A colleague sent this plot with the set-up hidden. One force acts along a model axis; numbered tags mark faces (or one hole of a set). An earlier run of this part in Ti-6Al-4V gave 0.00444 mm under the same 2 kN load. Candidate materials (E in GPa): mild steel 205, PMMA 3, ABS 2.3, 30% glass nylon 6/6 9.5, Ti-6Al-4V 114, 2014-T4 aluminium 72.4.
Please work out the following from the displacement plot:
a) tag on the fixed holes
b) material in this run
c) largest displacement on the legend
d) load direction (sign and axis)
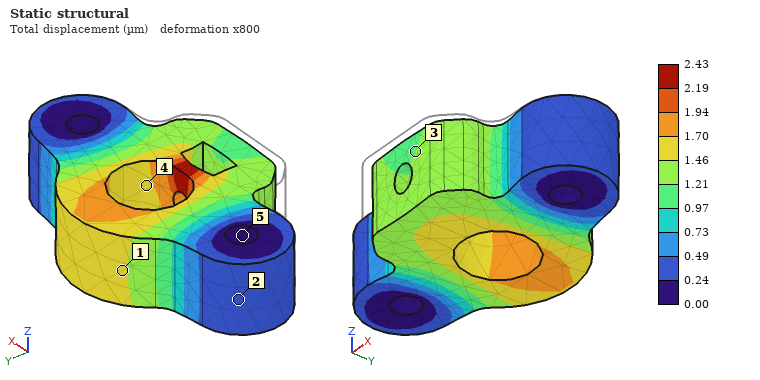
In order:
5
mild steel
2.43 µm
+Y
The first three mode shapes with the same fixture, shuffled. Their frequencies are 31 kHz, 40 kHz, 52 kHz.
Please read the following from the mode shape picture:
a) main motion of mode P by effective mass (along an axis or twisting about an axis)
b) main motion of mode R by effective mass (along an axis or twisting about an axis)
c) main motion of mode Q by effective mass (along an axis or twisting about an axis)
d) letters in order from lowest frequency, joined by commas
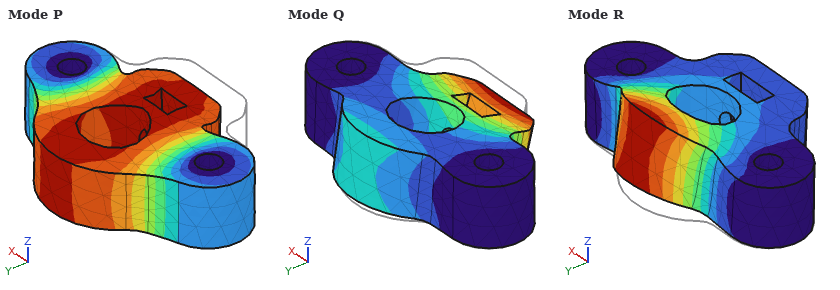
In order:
along Y
along Z
along Z
Q, R, P
